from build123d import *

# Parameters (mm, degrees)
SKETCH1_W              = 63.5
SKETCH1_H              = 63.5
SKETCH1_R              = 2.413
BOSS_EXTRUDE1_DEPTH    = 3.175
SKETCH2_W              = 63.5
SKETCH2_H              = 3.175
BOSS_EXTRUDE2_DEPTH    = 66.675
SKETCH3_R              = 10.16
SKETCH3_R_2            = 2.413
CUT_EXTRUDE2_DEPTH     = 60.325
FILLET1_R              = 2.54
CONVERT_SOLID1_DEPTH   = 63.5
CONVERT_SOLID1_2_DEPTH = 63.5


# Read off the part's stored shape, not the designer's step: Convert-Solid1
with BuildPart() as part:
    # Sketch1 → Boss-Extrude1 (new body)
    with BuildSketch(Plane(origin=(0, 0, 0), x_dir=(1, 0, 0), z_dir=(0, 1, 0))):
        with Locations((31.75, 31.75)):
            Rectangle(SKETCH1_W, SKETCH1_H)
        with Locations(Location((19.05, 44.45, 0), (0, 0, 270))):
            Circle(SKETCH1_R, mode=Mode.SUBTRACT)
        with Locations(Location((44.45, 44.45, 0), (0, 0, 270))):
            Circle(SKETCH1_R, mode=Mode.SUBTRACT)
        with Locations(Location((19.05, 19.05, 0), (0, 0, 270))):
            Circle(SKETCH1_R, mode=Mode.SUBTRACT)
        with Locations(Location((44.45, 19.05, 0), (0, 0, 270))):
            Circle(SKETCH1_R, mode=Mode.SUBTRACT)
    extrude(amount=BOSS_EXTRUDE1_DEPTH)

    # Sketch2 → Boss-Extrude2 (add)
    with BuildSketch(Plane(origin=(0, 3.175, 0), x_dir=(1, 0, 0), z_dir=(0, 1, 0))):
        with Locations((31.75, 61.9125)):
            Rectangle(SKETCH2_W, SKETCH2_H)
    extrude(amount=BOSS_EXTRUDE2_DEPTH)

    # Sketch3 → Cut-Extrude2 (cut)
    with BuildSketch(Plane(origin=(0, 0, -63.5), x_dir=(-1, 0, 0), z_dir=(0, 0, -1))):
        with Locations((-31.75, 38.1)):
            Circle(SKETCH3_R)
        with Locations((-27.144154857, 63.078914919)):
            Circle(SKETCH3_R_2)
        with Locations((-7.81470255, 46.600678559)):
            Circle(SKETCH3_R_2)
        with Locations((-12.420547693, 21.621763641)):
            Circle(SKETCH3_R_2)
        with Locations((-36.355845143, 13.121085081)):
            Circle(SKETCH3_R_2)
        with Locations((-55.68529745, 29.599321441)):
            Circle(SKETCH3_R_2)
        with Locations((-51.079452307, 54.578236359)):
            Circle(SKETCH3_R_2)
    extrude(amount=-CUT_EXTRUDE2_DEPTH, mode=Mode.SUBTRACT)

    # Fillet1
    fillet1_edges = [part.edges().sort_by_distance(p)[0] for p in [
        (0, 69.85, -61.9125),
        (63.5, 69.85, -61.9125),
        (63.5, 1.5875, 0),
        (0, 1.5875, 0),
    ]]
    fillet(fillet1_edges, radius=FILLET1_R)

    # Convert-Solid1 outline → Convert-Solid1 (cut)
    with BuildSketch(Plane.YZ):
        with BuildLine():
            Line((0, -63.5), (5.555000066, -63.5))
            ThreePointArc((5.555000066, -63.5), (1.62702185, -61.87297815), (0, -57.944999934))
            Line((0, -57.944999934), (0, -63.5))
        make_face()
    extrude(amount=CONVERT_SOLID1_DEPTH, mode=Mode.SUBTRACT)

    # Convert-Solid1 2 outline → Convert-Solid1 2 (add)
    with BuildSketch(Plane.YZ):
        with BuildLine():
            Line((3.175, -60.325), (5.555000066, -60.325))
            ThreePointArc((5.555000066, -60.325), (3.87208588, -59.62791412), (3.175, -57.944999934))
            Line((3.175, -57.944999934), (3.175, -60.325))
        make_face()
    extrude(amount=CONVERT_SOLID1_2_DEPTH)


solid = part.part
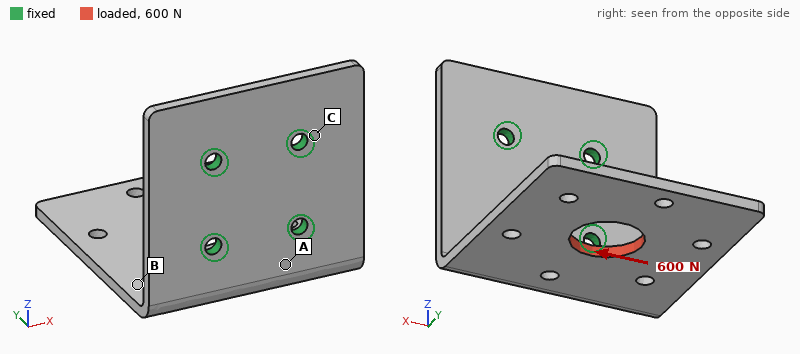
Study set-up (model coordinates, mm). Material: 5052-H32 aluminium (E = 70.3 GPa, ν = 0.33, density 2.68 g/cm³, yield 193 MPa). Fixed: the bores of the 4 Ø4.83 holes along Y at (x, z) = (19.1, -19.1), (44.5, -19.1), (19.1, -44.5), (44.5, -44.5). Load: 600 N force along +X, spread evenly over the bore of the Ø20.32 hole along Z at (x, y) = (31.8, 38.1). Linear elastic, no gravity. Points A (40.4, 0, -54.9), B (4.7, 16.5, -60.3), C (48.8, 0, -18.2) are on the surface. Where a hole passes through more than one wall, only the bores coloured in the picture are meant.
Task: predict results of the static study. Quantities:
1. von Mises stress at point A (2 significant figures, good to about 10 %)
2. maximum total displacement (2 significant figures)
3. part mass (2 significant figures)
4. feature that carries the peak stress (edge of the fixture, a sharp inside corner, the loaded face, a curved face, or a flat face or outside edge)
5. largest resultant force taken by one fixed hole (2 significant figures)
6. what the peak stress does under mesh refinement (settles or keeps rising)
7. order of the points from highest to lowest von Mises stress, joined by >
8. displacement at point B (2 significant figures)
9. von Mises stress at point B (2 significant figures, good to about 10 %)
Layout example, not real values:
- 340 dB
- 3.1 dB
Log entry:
- 68 MPa
- 0.55 mm
- 65 g
- edge of the fixture
- 830 N
- keeps rising
- A > B > C
- 0.22 mm
- 38 MPa
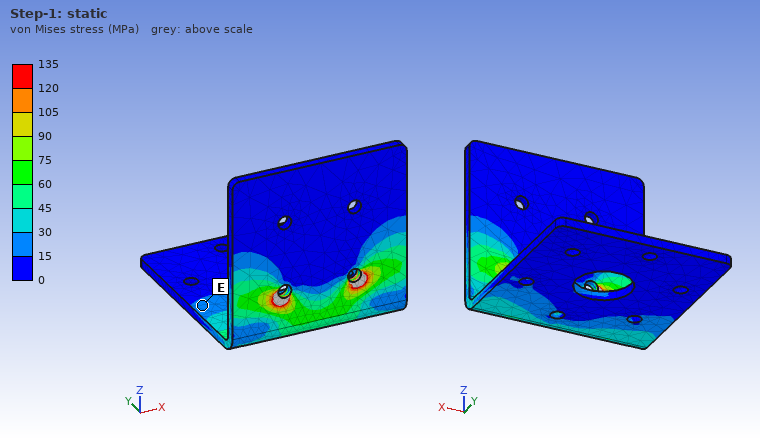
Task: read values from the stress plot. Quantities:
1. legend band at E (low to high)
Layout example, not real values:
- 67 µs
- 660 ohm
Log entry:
- 15 to 30 MPa
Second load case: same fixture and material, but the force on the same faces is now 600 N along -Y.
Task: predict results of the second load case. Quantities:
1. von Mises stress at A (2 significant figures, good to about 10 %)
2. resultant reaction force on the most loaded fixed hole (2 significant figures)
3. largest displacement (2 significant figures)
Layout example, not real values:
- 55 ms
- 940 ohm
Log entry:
- 40 MPa
- 350 N
- 0.53 mm
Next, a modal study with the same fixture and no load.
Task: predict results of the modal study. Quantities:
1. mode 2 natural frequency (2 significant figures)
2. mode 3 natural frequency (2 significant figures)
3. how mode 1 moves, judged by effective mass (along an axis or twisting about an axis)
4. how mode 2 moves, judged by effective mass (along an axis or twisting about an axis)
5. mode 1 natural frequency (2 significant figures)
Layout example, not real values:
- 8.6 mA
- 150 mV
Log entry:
- 1000 Hz
- 1400 Hz
- along Z
- along X
- 420 Hz
